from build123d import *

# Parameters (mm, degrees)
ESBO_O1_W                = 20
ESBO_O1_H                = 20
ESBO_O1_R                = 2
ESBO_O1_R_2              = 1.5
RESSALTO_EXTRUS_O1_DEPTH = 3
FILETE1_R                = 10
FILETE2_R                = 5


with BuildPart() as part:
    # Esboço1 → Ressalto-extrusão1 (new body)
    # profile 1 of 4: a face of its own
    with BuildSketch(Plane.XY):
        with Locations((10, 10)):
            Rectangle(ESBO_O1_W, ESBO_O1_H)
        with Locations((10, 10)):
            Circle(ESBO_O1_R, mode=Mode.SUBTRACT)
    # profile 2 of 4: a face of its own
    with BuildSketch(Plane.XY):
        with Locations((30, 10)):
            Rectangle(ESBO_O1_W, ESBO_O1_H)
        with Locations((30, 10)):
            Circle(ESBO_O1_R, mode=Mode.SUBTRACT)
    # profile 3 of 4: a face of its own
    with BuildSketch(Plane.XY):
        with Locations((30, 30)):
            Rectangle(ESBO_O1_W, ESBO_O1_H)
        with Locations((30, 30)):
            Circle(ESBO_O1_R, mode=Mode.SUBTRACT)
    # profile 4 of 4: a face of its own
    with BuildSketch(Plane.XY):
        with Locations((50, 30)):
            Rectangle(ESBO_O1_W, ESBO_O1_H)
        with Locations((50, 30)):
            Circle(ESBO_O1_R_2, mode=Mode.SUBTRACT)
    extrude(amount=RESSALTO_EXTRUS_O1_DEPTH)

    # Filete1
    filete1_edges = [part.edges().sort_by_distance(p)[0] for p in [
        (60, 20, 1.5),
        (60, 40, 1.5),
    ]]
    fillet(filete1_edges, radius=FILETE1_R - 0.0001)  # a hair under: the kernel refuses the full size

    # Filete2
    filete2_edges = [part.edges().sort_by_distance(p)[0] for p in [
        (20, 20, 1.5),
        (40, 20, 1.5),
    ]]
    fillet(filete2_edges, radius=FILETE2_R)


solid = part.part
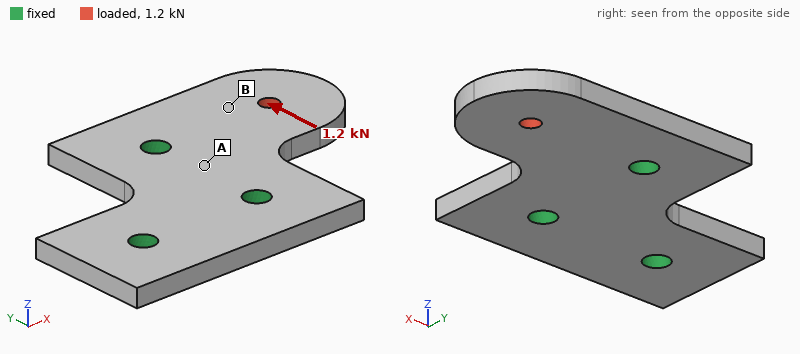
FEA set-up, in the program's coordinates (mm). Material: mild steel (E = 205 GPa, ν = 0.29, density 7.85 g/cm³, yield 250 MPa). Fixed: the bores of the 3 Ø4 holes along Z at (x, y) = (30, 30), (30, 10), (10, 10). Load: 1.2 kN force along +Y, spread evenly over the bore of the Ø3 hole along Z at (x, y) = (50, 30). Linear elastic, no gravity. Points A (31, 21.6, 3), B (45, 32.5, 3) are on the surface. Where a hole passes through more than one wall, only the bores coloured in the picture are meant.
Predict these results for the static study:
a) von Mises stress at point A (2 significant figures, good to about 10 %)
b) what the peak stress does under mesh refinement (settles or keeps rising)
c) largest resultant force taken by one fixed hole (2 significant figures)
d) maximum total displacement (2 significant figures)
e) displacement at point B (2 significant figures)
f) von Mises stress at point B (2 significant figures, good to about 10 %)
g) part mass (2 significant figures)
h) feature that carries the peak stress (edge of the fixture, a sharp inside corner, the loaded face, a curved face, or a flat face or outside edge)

18 MPa
keeps rising
1.2 kN
16 µm
7.7 µm
37 MPa
36 g
edge of the fixture
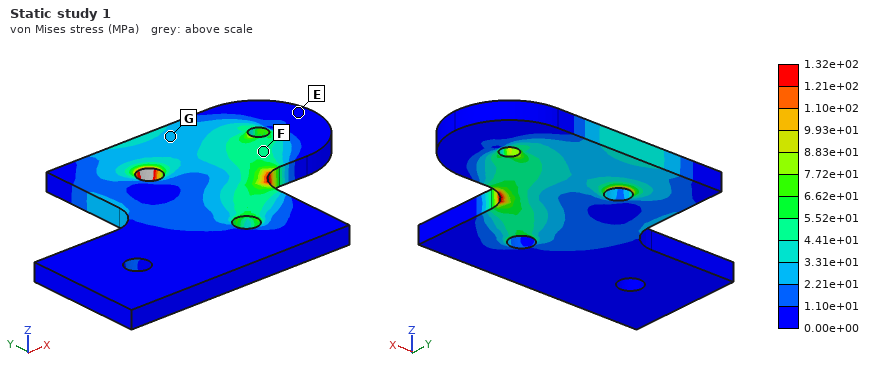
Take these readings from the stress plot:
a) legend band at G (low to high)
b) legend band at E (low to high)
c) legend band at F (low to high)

2.21e+01 to 3.31e+01 MPa
0.00e+00 to 1.10e+01 MPa
4.41e+01 to 5.52e+01 MPa
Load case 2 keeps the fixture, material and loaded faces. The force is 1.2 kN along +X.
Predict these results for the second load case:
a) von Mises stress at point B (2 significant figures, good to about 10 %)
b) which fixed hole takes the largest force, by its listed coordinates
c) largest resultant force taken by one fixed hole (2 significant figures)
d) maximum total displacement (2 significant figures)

30 MPa
(30, 30)
1.1 kN
3.6 µm
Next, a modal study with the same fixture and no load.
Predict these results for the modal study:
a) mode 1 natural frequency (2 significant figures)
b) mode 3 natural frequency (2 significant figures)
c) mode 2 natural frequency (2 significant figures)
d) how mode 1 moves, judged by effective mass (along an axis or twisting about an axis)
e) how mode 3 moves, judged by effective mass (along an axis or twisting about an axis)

3500 Hz
17 kHz
11 kHz
along Z
along Y
